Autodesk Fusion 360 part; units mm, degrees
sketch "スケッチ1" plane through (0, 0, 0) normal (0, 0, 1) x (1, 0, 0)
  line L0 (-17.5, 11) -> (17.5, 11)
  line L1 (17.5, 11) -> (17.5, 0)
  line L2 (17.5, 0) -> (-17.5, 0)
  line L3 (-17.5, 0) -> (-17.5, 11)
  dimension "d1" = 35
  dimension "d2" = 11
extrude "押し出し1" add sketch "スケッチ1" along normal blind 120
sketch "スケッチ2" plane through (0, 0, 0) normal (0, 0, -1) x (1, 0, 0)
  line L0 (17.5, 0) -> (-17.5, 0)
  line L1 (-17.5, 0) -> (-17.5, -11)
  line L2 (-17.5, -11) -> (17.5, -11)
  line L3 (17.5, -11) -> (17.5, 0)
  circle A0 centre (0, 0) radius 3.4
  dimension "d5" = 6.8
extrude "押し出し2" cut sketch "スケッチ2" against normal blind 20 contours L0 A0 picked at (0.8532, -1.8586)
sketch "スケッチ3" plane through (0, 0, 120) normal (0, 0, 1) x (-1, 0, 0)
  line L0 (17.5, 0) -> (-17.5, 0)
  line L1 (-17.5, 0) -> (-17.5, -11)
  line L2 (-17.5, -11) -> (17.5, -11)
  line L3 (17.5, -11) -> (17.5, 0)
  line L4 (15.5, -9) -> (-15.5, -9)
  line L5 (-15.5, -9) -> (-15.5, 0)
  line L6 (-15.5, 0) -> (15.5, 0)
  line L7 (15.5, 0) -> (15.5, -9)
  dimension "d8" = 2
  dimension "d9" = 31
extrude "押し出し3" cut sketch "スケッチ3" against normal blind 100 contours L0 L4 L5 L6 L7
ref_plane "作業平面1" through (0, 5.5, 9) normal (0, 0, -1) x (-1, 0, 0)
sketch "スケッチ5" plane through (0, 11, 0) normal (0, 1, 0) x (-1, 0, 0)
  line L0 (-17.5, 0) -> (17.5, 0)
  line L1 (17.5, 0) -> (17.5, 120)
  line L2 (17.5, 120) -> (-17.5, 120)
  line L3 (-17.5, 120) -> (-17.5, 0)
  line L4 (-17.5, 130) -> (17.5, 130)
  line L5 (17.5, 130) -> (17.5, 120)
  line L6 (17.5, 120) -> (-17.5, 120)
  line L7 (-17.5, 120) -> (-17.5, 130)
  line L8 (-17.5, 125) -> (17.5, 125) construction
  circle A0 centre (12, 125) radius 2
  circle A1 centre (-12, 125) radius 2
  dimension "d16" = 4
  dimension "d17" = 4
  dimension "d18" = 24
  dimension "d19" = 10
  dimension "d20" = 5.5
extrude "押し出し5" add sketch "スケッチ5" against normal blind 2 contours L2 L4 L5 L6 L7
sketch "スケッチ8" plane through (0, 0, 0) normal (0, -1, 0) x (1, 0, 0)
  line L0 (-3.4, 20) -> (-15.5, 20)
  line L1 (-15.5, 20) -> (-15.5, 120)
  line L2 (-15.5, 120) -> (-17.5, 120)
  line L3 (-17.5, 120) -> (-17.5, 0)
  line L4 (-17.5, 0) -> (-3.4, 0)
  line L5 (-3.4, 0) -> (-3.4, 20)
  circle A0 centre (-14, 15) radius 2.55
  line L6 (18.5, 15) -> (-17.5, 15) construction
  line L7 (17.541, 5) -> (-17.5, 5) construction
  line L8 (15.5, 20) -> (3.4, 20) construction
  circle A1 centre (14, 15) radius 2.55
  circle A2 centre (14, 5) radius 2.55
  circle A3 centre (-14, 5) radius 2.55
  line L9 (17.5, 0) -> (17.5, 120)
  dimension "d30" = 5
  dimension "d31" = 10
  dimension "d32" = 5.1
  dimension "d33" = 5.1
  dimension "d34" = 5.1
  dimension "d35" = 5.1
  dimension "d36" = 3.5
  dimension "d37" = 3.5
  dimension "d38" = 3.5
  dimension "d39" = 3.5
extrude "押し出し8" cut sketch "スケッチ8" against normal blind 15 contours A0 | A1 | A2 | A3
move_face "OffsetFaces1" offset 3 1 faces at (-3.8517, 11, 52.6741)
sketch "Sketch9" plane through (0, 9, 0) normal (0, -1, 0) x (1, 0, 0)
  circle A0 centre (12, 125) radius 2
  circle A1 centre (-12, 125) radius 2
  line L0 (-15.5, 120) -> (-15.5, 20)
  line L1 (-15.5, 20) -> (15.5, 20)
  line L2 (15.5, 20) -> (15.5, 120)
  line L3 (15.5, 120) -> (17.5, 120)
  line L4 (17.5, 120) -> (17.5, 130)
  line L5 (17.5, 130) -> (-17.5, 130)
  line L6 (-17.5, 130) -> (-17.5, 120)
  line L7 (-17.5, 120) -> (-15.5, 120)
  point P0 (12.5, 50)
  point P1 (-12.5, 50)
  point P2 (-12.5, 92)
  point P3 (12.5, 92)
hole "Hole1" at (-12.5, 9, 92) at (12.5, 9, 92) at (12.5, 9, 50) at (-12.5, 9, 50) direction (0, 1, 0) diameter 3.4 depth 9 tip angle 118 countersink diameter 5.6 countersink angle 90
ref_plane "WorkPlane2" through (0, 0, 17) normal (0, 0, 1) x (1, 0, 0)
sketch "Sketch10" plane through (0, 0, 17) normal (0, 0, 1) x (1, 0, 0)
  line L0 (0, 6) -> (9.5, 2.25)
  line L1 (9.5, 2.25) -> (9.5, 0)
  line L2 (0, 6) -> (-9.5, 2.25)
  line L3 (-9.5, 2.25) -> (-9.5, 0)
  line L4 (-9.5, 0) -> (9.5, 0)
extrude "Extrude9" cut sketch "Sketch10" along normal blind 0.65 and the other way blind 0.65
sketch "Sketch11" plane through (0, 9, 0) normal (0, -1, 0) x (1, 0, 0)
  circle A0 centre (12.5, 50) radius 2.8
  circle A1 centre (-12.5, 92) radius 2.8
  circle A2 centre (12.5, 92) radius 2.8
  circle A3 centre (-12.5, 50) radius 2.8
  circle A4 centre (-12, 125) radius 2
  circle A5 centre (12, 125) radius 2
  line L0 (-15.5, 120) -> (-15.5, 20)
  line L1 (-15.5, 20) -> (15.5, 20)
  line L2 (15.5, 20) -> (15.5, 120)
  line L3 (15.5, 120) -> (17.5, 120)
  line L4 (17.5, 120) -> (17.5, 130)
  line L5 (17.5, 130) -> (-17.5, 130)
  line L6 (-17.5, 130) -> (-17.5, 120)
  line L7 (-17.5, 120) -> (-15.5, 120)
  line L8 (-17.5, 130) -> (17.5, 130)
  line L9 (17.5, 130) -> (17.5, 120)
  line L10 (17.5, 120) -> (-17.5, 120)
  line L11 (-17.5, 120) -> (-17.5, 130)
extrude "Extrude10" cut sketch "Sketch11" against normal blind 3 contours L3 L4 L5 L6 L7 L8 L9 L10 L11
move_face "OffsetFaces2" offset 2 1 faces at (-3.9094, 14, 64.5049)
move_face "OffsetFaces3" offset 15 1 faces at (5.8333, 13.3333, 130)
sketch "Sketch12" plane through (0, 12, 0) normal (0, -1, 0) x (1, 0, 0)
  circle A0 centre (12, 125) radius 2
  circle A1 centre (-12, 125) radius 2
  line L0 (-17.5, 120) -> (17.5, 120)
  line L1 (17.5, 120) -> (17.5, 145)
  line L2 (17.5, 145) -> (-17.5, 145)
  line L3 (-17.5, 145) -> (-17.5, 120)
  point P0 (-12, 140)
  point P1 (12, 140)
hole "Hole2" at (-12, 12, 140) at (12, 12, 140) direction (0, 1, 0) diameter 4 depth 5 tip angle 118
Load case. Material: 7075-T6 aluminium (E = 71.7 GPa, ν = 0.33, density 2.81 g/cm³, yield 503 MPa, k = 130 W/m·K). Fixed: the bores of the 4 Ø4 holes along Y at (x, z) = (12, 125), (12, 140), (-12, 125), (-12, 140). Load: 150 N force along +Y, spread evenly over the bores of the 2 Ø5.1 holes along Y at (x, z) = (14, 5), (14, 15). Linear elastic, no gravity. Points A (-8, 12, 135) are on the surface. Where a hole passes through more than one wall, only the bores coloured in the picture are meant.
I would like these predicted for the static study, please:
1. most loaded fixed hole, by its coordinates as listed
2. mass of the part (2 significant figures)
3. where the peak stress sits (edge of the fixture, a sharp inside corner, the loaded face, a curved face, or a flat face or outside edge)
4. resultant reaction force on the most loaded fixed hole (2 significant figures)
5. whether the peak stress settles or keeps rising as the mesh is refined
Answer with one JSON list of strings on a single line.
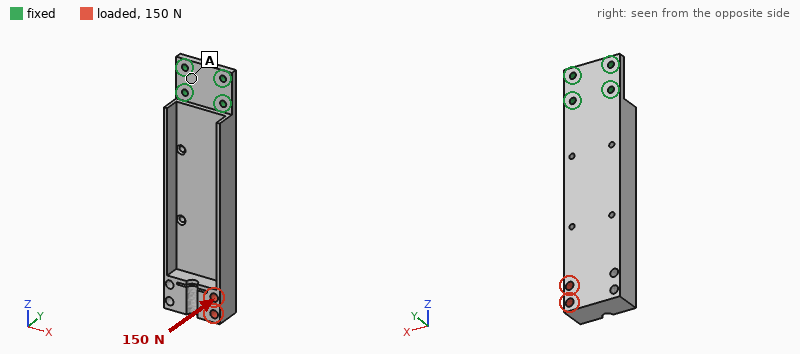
["(12, 125)", "110 g", "edge of the fixture", "340 N", "keeps rising"]
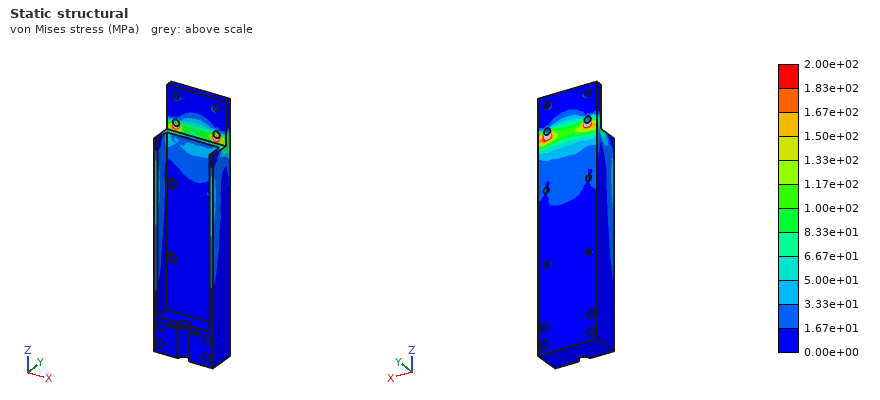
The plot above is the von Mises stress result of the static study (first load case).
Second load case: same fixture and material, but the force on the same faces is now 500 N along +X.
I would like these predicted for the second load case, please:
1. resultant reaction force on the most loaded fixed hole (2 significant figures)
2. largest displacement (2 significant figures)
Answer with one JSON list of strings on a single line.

["2.1 kN", "0.20 mm"]
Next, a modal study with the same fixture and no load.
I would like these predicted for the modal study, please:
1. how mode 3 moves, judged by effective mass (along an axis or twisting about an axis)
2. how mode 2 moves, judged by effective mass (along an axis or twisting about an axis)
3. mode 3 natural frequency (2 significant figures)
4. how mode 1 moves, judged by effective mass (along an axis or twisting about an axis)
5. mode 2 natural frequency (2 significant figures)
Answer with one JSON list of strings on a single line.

["twisting about Z", "along X", "1800 Hz", "along Y", "1300 Hz"]
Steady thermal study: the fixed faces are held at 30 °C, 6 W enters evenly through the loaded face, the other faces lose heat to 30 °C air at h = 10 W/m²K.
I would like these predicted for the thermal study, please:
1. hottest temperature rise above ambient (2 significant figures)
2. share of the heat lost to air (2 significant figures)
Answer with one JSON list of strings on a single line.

["18 K", "26 %"]
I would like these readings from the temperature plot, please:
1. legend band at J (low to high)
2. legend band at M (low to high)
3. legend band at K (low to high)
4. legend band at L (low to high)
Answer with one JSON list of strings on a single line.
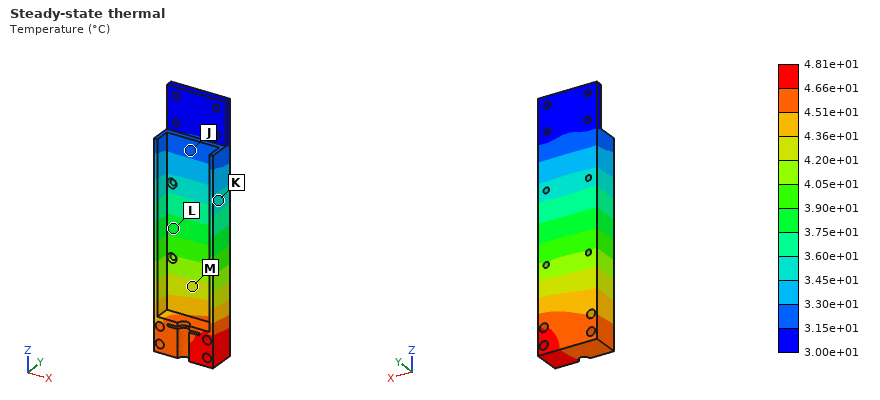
["3.15e+01 to 3.30e+01 °C", "4.20e+01 to 4.36e+01 °C", "3.45e+01 to 3.60e+01 °C", "3.75e+01 to 3.90e+01 °C"]
